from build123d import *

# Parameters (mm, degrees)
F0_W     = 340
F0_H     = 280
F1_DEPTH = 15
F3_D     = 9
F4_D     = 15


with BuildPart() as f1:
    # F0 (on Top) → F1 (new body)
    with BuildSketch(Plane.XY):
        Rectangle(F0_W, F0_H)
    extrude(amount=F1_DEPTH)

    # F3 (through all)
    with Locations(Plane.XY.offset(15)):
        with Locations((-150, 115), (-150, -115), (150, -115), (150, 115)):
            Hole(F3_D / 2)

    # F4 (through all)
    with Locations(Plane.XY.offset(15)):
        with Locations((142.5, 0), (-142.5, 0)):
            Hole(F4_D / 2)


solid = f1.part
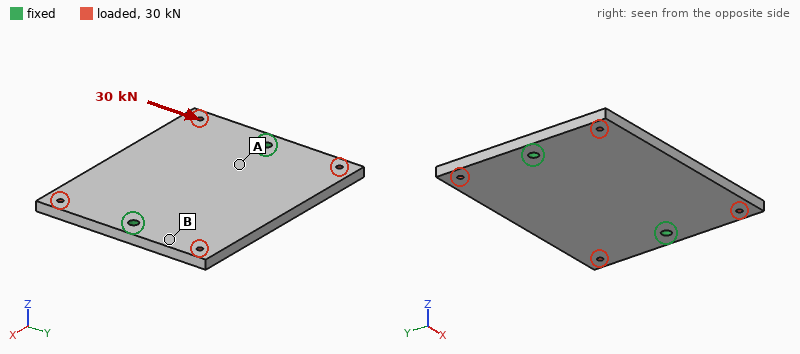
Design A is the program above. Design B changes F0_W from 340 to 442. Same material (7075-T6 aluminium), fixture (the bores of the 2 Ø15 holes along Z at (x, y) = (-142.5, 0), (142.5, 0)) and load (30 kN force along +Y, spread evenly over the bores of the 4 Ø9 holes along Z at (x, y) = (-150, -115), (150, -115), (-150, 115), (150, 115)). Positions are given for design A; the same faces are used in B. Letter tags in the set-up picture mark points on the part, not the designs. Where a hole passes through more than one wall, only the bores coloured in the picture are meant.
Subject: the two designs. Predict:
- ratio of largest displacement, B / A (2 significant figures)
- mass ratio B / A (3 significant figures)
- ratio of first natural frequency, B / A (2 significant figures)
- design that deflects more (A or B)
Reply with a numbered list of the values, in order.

1. 0.87
2. 1.30
3. 1.0
4. A
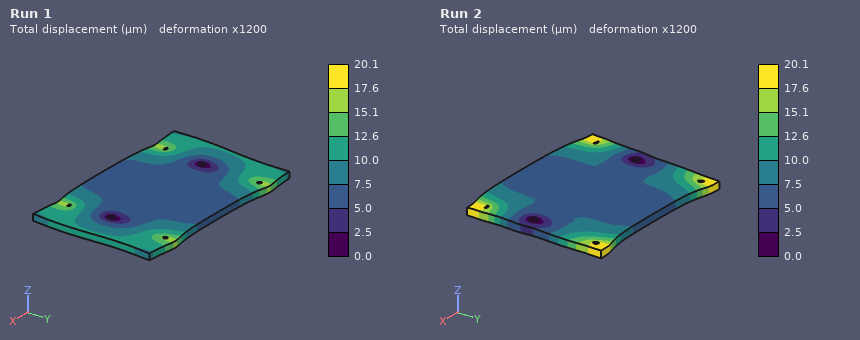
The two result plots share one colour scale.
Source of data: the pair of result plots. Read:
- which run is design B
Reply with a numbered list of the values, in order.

1. Run 1
